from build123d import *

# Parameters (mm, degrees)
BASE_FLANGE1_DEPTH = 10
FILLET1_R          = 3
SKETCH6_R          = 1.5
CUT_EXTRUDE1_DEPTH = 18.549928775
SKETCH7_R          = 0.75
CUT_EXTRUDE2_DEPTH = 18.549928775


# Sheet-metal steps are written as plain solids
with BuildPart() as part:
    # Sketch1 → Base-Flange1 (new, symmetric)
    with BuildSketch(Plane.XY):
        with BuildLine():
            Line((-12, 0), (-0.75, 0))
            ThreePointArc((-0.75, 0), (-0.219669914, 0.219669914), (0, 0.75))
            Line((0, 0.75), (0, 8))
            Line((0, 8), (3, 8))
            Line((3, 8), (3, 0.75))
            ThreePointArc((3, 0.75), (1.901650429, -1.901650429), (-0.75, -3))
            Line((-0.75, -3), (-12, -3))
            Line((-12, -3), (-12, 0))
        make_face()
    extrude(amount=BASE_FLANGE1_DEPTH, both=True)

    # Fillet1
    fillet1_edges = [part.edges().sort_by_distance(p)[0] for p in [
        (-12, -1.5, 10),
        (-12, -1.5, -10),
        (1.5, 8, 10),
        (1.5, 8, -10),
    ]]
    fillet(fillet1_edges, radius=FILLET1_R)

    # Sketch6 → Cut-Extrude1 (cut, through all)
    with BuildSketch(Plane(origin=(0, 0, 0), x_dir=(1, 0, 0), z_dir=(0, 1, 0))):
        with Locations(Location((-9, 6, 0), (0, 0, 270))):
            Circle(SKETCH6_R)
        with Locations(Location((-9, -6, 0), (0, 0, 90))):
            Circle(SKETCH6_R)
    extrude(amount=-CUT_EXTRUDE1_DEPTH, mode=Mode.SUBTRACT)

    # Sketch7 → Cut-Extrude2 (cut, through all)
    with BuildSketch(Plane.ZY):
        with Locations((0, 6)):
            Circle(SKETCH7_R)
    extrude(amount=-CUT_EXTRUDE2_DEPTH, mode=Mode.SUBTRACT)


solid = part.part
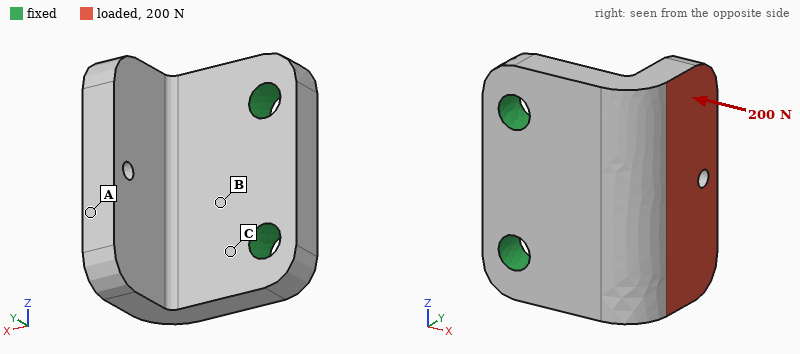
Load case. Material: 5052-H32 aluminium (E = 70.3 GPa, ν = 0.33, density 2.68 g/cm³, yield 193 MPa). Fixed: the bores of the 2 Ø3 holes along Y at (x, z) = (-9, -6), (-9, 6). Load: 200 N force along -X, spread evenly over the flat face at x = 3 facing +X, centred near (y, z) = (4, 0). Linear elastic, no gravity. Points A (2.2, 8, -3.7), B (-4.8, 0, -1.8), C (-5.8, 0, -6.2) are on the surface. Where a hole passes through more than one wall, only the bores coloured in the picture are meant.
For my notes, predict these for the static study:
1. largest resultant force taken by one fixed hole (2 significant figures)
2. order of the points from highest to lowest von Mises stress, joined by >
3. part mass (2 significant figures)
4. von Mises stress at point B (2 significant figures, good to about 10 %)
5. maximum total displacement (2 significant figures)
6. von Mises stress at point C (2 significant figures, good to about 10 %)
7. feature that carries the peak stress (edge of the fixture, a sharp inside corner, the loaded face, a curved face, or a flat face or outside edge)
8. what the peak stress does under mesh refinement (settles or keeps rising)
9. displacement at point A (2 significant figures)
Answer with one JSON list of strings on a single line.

["100 N", "C > B > A", "3.4 g", "34 MPa", "46 µm", "48 MPa", "edge of the fixture", "keeps rising", "44 µm"]
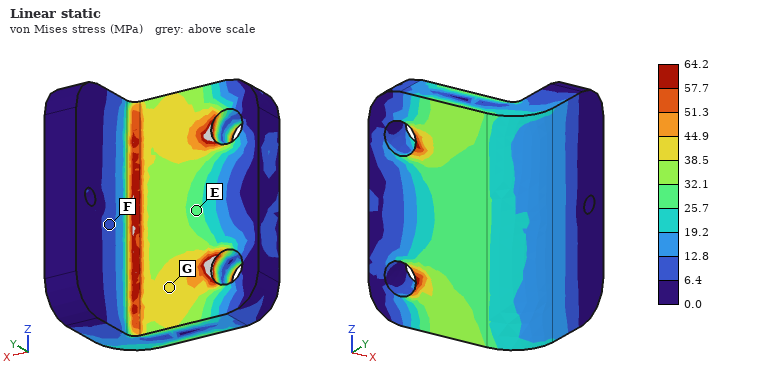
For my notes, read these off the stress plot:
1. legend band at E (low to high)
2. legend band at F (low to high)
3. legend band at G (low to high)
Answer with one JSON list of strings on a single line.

["25.7 to 32.1 MPa", "6.4 to 12.8 MPa", "38.5 to 44.9 MPa"]
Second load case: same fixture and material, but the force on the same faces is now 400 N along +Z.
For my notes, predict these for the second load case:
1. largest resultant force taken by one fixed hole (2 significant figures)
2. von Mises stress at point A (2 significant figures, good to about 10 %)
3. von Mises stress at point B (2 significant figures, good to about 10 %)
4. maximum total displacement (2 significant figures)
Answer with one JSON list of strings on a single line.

["420 N", "7.5 MPa", "44 MPa", "28 µm"]
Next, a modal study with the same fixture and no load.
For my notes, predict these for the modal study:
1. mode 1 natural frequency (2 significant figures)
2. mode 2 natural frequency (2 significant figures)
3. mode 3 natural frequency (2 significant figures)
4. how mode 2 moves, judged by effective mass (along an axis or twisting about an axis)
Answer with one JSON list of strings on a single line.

["9000 Hz", "15 kHz", "26 kHz", "along Z"]
